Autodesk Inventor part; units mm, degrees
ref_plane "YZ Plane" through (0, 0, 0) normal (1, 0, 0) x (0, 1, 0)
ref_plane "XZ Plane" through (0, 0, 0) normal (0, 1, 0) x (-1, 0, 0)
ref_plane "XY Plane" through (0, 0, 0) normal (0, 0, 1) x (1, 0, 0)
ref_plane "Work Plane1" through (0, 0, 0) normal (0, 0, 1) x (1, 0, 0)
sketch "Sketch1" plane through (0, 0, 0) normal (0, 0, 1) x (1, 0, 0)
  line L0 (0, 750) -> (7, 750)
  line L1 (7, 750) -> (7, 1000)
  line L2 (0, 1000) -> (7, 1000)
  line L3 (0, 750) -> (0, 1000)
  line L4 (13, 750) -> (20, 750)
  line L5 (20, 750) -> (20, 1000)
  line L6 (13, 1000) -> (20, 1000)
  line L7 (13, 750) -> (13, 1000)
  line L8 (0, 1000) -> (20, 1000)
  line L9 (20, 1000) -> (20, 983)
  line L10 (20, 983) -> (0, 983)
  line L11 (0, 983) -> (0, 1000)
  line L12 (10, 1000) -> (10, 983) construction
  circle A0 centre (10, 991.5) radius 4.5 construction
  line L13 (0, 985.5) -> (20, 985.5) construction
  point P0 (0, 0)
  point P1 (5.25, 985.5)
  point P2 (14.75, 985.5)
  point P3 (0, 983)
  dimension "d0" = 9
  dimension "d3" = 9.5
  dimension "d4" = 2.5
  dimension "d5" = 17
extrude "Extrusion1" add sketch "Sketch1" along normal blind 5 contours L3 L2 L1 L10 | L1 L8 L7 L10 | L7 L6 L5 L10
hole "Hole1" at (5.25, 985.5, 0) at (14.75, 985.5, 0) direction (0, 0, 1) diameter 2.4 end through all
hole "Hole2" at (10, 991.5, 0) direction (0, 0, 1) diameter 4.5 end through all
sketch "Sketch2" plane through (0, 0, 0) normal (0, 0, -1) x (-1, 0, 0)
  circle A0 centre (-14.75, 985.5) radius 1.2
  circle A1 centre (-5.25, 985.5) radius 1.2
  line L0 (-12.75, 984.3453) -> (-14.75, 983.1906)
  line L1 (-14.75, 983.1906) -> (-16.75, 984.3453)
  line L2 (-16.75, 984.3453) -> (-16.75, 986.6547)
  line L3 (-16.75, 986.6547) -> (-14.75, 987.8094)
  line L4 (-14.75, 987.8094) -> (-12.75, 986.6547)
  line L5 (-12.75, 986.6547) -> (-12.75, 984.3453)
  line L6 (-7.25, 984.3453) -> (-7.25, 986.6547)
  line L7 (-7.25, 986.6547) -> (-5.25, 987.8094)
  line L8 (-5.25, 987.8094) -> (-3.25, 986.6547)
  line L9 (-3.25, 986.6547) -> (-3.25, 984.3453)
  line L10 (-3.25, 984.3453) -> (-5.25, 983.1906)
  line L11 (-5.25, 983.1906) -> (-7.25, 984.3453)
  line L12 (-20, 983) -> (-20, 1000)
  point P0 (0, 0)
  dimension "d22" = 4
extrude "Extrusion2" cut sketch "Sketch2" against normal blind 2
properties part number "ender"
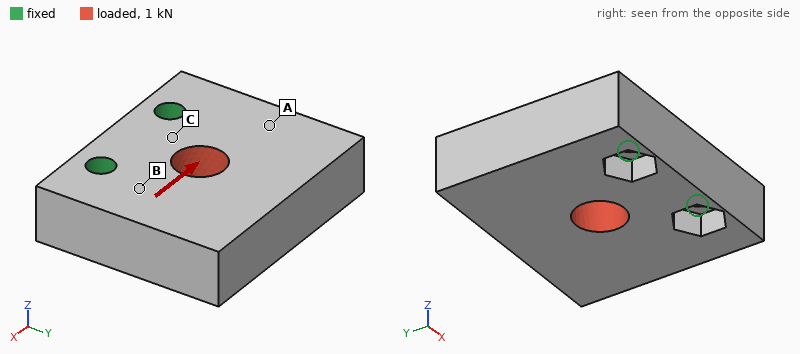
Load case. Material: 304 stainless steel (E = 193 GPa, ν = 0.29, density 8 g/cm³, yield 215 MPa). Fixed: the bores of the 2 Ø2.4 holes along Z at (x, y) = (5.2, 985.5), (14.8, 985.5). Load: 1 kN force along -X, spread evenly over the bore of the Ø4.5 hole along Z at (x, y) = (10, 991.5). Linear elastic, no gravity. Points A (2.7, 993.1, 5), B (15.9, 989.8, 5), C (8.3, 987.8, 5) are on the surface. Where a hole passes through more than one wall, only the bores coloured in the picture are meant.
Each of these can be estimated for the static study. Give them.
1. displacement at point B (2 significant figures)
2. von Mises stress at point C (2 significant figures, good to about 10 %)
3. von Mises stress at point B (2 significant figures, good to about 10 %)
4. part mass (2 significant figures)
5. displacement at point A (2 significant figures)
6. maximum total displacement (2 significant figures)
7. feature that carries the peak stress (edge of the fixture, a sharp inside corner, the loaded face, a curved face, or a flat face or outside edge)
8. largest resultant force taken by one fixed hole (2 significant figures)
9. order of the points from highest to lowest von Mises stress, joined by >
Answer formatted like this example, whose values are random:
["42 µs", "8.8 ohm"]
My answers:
["1.4 µm", "37 MPa", "20 MPa", "12 g", "2.4 µm", "3.7 µm", "edge of the fixture", "700 N", "C > B > A"]
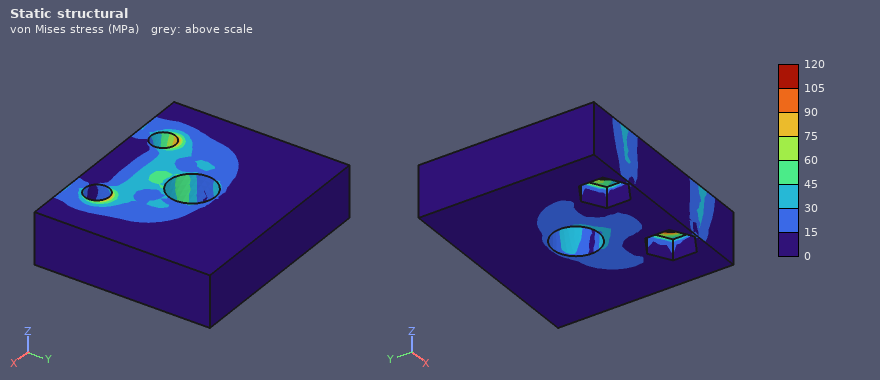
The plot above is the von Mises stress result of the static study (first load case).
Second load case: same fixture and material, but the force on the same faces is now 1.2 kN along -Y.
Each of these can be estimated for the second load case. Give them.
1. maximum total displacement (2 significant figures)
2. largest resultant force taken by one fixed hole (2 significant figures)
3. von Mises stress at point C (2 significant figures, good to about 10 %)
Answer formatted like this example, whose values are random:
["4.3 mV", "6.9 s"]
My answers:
["3.8 µm", "610 N", "14 MPa"]
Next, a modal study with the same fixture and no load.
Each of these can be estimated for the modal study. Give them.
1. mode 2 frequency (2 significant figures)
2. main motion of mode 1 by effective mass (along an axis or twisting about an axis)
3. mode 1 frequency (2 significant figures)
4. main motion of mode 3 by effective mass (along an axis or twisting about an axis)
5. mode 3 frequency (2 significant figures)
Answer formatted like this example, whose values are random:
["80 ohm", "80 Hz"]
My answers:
["22 kHz", "along Z", "11 kHz", "along X", "26 kHz"]
